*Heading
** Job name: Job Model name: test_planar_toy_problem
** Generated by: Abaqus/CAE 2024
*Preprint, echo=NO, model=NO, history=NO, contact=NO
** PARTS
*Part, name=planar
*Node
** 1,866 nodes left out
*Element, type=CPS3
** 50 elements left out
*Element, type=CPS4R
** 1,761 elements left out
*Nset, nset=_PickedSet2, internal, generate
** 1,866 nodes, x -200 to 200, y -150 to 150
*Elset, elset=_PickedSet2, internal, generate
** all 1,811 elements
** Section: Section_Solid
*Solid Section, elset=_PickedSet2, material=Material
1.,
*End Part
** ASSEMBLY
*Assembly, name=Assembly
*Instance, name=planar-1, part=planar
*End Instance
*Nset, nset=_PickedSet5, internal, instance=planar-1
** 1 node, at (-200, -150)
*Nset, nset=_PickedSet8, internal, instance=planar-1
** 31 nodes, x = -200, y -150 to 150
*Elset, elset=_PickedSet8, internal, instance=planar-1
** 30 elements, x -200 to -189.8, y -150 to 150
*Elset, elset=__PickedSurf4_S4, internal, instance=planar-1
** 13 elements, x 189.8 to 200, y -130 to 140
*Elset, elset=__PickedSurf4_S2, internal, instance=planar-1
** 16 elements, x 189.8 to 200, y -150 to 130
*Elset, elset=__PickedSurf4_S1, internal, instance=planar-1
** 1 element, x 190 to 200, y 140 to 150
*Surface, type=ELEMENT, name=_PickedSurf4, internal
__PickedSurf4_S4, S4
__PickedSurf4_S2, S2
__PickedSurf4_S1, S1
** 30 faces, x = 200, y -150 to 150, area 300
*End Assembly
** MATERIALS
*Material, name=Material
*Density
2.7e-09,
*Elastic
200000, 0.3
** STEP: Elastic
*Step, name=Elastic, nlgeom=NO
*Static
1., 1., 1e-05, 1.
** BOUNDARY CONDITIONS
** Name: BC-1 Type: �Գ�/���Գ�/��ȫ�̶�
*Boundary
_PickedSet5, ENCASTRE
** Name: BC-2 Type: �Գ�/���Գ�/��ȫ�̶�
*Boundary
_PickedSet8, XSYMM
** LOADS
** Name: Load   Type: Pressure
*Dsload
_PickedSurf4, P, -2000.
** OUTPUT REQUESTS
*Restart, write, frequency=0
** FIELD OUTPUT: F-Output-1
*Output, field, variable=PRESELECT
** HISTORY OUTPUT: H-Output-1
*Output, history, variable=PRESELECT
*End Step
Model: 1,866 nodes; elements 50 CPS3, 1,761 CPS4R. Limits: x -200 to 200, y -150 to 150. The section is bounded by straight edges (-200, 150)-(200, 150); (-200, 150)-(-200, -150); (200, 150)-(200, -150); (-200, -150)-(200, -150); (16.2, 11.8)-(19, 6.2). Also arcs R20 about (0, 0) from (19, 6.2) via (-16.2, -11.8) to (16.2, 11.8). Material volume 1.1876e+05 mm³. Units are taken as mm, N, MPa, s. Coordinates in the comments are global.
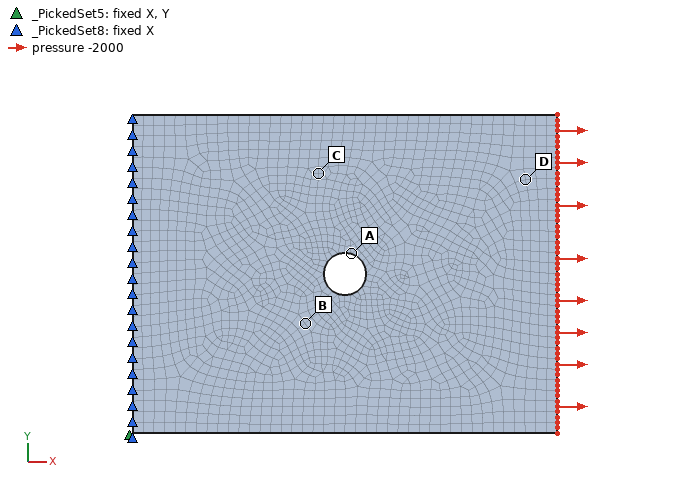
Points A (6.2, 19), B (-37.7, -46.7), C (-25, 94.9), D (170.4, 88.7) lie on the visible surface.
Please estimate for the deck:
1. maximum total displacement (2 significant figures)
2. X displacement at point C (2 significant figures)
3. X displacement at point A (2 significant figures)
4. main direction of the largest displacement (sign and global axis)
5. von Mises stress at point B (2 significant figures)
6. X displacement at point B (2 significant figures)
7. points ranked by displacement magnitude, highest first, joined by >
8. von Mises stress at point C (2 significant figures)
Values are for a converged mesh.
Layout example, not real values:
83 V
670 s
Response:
4.2 mm
1.8 mm
2.3 mm
+X
2400 MPa
1.6 mm
D > A > C > B
2100 MPa
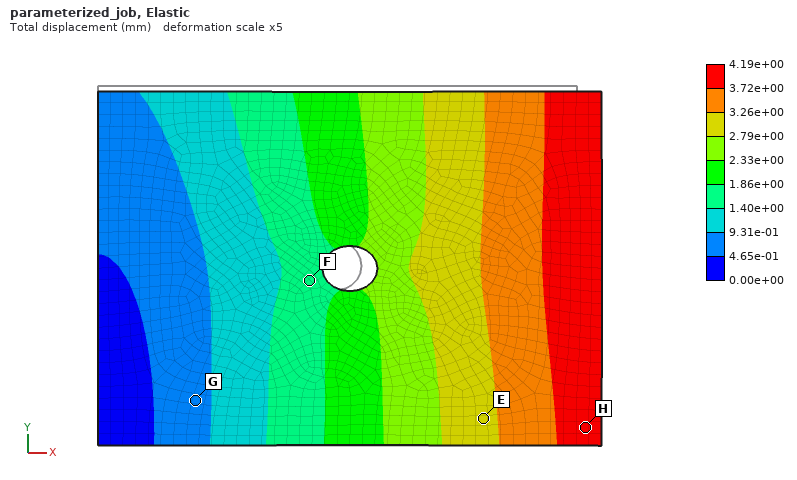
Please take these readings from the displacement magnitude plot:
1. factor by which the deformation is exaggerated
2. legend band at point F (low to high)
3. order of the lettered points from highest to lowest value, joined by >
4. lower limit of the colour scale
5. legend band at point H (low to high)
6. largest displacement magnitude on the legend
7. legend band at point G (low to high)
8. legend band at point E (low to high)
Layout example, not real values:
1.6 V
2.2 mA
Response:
5
1.40e+00 to 1.86e+00 mm
H > E > F > G
0.00e+00 mm
3.72e+00 to 4.19e+00 mm
4.19e+00 mm
4.65e-01 to 9.31e-01 mm
2.79e+00 to 3.26e+00 mm
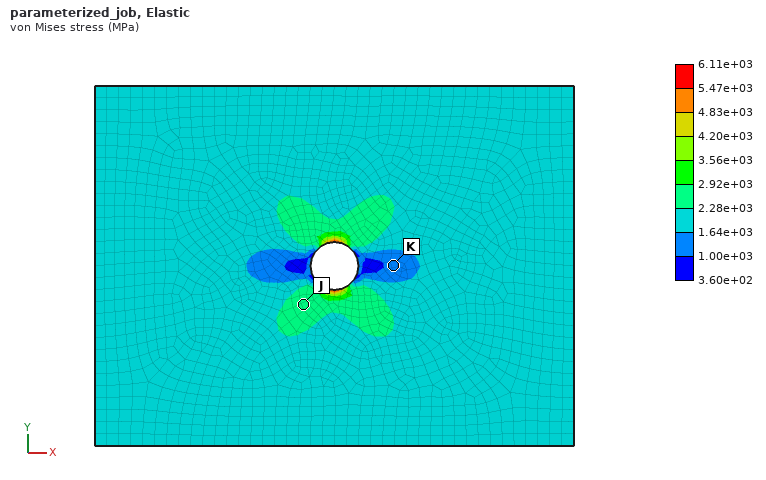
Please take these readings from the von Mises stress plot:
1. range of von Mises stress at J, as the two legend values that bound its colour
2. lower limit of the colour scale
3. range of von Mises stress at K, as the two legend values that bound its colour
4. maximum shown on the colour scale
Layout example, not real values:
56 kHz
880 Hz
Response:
2.28e+03 to 2.92e+03 MPa
3.60e+02 MPa
1.00e+03 to 1.64e+03 MPa
6.11e+03 MPa
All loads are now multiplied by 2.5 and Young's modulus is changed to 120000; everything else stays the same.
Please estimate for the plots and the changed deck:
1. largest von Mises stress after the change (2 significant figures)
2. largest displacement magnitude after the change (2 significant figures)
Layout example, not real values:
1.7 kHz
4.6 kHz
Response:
15000 MPa
17 mm
